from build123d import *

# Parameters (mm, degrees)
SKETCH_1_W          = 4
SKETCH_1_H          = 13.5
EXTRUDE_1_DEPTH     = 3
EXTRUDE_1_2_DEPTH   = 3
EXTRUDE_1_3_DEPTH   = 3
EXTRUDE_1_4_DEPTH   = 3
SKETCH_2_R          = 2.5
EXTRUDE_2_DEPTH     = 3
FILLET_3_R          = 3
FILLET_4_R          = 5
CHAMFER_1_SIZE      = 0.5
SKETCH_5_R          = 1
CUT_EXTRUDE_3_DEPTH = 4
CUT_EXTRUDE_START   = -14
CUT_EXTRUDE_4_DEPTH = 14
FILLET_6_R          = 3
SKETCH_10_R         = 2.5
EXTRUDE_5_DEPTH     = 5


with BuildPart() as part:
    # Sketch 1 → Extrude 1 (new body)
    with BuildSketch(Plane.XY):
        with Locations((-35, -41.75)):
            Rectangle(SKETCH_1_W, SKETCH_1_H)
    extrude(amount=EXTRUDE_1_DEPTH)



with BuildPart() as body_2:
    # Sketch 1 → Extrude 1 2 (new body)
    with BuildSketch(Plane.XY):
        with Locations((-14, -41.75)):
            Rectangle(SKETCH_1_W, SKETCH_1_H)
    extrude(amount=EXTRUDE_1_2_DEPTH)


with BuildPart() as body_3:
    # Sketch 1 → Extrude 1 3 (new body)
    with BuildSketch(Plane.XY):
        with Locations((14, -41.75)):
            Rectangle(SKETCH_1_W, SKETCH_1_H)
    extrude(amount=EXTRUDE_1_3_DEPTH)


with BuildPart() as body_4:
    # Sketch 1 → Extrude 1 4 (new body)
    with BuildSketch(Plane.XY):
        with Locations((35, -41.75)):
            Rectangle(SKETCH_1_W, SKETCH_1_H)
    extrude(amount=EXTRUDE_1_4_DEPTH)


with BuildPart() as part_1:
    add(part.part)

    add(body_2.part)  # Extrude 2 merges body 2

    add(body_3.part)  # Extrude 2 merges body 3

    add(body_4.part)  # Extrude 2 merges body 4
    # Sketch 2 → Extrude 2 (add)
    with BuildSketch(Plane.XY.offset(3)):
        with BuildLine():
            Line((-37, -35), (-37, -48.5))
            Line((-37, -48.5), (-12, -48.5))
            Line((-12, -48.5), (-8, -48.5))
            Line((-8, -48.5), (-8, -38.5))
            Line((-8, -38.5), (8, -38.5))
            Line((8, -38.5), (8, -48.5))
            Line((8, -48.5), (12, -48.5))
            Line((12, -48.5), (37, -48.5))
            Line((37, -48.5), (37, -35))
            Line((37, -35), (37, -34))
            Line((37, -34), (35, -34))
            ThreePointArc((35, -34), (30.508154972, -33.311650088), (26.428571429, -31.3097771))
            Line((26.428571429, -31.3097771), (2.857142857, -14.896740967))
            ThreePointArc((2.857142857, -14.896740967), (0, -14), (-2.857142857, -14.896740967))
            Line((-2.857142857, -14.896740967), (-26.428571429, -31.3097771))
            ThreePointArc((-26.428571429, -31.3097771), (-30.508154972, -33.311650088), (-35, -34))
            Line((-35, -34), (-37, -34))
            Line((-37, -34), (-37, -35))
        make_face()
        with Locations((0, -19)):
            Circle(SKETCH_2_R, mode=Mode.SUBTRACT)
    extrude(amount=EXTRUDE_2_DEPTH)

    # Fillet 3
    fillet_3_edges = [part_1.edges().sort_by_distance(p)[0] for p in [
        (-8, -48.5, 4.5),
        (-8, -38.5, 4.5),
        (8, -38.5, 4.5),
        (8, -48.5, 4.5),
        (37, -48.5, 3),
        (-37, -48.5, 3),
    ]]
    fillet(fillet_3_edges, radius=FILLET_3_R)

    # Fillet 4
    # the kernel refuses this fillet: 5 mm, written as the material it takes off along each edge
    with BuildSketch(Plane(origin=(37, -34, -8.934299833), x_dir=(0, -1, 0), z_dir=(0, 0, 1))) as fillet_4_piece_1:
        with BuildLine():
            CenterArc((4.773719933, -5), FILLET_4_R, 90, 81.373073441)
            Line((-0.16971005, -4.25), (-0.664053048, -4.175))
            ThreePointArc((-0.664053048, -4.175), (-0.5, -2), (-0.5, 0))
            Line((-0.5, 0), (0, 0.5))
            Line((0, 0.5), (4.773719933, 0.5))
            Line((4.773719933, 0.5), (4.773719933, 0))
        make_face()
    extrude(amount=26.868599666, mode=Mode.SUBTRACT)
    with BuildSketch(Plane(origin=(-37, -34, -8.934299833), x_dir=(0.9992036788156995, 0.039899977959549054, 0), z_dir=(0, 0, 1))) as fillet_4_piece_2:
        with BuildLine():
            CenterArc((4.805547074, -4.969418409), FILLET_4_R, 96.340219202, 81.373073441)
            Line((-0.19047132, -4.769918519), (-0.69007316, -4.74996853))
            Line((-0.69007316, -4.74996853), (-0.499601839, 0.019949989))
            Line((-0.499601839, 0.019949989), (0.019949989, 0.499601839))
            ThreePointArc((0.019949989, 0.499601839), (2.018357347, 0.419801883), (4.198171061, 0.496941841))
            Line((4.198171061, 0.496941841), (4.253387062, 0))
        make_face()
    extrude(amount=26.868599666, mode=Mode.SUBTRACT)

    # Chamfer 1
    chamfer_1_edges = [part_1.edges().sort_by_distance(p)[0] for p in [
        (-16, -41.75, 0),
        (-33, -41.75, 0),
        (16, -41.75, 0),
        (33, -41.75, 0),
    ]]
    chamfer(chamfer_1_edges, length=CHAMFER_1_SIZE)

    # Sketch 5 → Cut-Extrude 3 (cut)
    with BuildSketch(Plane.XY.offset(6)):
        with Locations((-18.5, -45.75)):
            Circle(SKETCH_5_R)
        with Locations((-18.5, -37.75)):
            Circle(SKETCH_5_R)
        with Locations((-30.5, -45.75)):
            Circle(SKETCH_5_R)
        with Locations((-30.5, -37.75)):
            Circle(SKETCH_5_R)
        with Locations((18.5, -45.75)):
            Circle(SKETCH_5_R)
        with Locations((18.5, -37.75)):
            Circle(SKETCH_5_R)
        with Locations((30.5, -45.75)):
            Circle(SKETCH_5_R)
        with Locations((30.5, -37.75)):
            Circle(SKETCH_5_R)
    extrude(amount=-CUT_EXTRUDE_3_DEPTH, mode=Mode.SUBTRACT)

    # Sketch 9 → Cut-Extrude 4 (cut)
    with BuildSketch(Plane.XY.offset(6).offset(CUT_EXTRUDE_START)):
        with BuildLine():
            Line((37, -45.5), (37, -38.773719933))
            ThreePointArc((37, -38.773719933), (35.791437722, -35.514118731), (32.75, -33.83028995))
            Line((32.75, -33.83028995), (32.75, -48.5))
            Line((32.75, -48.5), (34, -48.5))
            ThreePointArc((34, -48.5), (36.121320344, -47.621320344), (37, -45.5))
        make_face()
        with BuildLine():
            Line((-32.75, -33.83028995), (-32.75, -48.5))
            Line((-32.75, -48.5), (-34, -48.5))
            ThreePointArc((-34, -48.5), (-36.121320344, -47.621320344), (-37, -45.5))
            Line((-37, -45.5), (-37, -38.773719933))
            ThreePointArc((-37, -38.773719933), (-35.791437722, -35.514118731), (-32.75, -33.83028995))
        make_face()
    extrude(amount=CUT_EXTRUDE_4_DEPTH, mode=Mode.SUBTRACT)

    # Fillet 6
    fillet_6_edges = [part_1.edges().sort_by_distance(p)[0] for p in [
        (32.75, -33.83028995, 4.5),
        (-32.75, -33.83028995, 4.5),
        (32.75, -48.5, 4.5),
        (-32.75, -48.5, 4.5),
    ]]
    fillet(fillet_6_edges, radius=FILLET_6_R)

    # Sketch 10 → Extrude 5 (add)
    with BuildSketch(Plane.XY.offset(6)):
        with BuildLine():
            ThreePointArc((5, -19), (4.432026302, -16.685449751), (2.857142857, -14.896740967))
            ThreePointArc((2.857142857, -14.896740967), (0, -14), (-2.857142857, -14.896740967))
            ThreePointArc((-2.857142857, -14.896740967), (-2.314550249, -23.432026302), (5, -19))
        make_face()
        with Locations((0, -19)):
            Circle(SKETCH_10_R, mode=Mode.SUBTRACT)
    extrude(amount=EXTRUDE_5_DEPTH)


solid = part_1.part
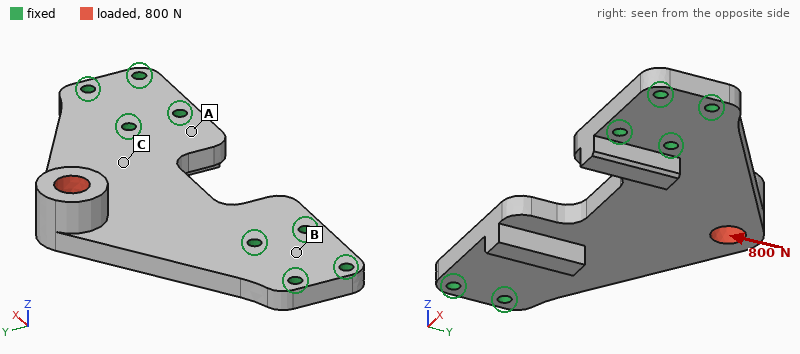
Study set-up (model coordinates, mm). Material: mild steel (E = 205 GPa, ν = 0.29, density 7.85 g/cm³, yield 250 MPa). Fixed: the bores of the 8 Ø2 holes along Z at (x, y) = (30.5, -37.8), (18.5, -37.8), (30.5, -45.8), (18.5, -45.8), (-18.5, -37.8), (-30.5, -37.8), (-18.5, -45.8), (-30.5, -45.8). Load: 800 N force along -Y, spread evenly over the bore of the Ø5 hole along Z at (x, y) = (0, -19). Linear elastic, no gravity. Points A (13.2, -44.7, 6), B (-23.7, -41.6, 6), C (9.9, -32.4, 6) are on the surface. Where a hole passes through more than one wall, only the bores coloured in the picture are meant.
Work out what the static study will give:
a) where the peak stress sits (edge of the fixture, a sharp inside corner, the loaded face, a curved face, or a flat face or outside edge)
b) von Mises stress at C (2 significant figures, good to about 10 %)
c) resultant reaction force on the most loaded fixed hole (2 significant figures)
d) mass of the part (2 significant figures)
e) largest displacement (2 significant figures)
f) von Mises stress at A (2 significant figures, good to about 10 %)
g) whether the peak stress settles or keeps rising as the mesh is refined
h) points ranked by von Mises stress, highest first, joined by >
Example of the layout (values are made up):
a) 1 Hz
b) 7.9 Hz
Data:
a) edge of the fixture
b) 42 MPa
c) 300 N
d) 37 g
e) 44 µm
f) 13 MPa
g) keeps rising
h) C > A > B
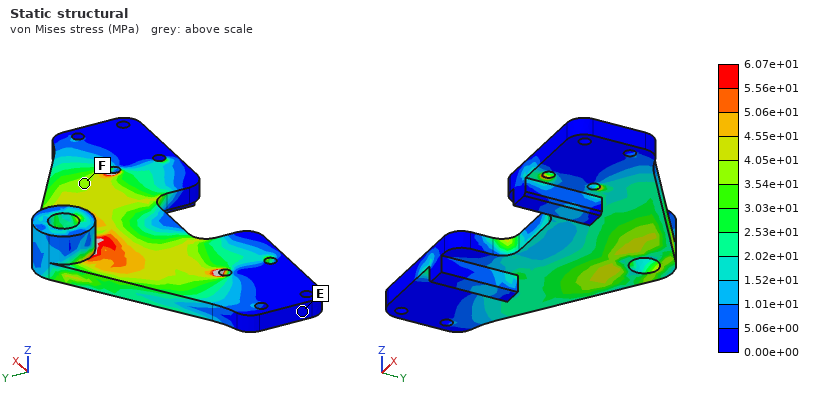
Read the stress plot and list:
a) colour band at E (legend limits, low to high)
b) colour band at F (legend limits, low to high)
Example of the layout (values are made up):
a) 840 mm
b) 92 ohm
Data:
a) 0.00e+00 to 5.06e+00 MPa
b) 3.54e+01 to 4.05e+01 MPa
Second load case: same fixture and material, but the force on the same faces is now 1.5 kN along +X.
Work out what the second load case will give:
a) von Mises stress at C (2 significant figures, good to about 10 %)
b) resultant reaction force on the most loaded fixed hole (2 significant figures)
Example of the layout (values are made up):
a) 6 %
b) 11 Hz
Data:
a) 38 MPa
b) 560 N
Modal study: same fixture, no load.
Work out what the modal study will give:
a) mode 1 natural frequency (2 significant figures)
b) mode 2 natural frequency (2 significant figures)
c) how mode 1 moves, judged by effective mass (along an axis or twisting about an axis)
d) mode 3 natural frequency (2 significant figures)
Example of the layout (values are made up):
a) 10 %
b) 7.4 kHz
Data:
a) 4400 Hz
b) 13 kHz
c) along Z
d) 14 kHz
